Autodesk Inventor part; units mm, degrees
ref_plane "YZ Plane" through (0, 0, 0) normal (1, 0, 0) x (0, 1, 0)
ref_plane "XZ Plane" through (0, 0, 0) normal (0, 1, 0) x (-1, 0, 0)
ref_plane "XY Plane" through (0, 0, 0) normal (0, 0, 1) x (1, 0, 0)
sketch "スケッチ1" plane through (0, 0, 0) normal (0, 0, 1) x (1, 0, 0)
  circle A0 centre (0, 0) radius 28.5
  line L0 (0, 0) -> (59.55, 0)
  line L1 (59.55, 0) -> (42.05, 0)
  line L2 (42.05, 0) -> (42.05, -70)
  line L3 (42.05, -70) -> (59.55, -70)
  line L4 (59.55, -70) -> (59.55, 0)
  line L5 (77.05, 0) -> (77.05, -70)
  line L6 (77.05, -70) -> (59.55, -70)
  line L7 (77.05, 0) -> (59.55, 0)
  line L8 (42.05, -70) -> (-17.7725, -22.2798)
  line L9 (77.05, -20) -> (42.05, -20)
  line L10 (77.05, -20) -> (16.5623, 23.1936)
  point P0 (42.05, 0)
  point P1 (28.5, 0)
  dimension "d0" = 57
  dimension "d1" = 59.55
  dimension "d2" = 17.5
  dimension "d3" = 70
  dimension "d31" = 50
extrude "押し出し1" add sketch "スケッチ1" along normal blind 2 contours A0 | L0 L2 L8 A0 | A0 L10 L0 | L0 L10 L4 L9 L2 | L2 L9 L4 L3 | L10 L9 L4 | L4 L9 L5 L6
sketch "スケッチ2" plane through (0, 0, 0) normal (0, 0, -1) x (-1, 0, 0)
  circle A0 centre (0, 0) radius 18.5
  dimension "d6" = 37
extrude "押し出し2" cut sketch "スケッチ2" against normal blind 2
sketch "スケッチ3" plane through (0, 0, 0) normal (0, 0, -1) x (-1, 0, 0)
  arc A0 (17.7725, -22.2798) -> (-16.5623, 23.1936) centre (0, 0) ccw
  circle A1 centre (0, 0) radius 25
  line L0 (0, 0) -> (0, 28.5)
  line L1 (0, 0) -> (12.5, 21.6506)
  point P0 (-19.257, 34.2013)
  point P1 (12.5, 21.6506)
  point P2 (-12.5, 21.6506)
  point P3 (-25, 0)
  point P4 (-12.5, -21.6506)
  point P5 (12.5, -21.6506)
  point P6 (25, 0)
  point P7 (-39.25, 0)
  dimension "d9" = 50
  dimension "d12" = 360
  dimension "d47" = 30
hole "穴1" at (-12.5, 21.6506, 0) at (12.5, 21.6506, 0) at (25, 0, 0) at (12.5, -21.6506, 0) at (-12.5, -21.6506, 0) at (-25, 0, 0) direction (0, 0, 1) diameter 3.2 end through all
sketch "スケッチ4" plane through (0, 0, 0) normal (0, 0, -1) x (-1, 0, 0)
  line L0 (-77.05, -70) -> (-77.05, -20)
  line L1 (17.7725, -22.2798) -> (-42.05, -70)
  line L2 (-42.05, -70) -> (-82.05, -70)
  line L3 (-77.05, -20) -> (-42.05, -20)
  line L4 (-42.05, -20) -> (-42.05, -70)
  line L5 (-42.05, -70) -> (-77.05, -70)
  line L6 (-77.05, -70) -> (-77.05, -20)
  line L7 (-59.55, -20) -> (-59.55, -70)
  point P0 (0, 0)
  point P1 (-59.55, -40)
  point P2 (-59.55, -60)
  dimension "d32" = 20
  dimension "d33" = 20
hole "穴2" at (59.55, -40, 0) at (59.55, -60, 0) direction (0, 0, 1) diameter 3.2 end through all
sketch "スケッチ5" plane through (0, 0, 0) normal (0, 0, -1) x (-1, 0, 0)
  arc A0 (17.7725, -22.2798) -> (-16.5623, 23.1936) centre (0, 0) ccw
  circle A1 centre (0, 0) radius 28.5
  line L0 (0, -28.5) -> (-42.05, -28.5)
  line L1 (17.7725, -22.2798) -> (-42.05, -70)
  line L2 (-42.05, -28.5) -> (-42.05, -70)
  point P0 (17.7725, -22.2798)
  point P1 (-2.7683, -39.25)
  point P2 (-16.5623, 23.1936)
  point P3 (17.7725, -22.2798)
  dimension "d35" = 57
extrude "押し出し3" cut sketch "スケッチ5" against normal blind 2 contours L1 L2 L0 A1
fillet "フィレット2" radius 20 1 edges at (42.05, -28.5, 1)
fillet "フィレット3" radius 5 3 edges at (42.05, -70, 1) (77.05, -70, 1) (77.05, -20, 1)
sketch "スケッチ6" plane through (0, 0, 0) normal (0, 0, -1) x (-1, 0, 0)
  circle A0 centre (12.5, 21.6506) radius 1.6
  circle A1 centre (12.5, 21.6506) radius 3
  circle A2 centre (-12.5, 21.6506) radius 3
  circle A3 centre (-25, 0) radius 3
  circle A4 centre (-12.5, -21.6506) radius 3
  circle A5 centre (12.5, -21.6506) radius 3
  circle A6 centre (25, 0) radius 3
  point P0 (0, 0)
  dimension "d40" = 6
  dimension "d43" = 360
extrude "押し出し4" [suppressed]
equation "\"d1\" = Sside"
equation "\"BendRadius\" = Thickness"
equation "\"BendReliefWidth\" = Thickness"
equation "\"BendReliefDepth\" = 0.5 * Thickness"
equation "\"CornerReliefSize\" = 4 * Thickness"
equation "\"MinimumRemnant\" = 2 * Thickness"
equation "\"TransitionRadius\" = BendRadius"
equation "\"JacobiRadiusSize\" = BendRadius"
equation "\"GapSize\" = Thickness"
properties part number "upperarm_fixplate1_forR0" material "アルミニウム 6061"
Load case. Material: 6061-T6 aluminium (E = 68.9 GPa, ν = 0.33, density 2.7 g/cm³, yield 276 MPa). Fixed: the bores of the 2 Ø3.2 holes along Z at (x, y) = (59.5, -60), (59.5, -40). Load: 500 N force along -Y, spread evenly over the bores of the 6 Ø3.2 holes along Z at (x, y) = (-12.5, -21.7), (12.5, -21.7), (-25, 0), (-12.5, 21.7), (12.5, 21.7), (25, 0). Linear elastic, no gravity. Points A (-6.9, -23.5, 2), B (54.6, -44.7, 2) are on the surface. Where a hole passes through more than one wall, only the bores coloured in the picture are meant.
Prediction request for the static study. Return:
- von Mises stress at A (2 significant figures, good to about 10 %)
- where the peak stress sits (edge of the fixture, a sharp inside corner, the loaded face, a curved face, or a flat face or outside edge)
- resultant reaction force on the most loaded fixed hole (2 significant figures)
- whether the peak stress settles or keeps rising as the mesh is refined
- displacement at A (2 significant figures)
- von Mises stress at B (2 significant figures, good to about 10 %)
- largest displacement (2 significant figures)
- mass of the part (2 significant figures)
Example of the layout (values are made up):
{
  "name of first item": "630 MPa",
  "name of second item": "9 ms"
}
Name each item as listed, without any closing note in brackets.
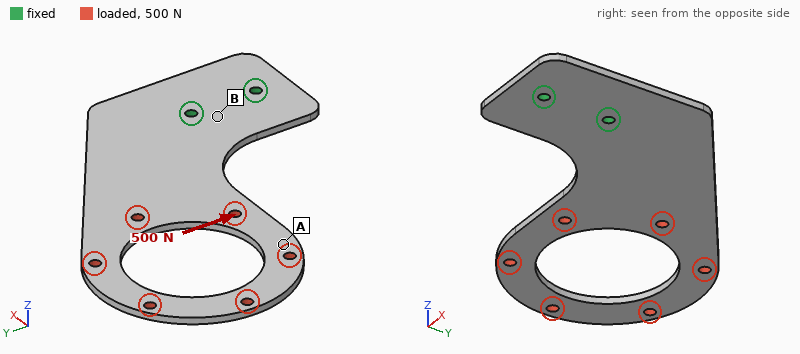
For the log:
{
  "von Mises stress at A": "18 MPa",
  "where the peak stress sits": "edge of the fixture",
  "resultant reaction force on the most loaded fixed hole": "1.4 kN",
  "whether the peak stress settles or keeps rising as the mesh is refined": "keeps rising",
  "displacement at A": "0.25 mm",
  "von Mises stress at B": "50 MPa",
  "largest displacement": "0.39 mm",
  "mass of the part": "24 g"
}
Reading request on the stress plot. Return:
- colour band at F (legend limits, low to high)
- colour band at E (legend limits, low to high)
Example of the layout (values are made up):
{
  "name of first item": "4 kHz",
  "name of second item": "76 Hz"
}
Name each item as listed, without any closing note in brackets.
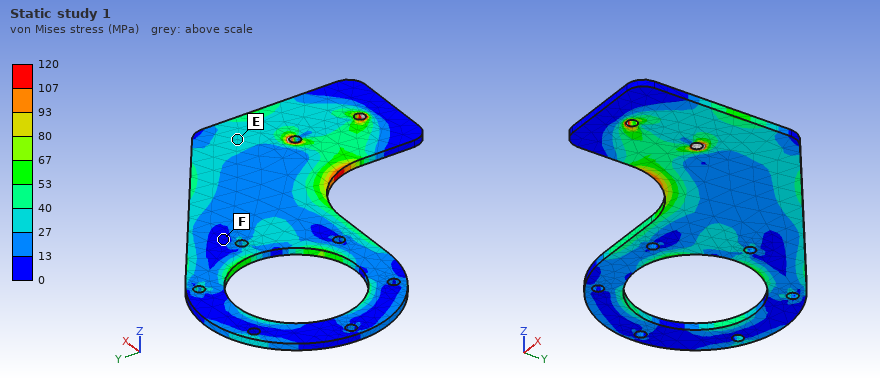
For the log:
{
  "colour band at F": "0 to 13 MPa",
  "colour band at E": "27 to 40 MPa"
}
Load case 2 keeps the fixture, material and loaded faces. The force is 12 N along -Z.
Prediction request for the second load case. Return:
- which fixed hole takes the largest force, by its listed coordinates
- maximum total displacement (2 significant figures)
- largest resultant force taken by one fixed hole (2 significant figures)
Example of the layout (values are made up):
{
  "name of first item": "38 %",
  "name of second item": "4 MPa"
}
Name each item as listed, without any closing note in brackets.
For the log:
{
  "which fixed hole takes the largest force, by its listed coordinates": "(59.5, -40)",
  "maximum total displacement": "1.6 mm",
  "largest resultant force taken by one fixed hole": "24 N"
}
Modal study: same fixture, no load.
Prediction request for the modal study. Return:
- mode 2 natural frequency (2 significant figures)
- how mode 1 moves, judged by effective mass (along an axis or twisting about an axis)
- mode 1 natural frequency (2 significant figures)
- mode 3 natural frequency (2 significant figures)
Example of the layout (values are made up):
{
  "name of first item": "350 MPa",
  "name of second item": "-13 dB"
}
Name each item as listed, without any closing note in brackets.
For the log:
{
  "mode 2 natural frequency": "550 Hz",
  "how mode 1 moves, judged by effective mass": "along Z",
  "mode 1 natural frequency": "180 Hz",
  "mode 3 natural frequency": "900 Hz"
}
